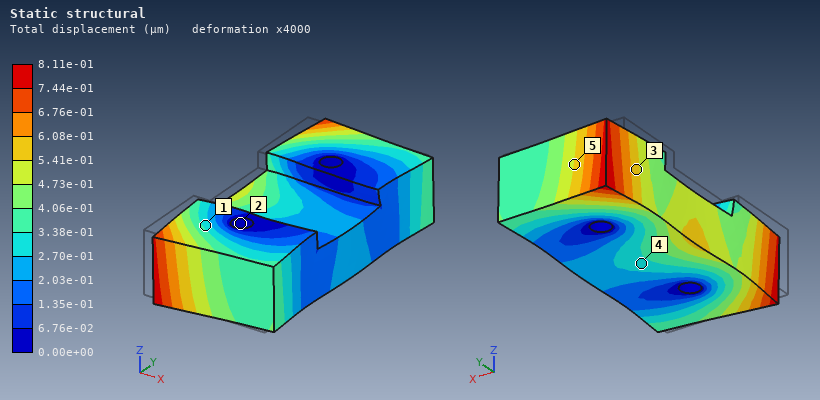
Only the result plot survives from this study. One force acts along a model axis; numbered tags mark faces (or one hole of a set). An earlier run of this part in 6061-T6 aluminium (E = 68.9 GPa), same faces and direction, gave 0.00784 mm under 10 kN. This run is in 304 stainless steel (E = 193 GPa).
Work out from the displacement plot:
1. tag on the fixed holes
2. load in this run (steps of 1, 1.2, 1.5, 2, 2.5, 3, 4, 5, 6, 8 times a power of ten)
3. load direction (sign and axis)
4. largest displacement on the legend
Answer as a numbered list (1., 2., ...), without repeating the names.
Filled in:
1. 2
2. 3 kN
3. +X
4. 8.11e-01 µm
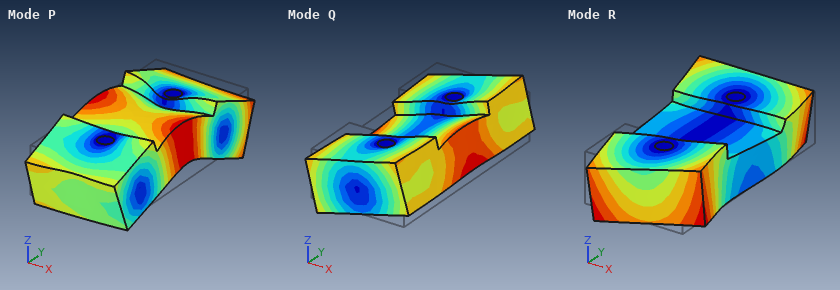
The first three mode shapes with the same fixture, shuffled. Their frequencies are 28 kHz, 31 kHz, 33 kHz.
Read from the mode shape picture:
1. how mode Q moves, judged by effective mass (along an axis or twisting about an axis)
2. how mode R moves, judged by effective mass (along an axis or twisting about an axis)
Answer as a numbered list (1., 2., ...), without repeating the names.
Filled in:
1. twisting about Y
2. twisting about Z
